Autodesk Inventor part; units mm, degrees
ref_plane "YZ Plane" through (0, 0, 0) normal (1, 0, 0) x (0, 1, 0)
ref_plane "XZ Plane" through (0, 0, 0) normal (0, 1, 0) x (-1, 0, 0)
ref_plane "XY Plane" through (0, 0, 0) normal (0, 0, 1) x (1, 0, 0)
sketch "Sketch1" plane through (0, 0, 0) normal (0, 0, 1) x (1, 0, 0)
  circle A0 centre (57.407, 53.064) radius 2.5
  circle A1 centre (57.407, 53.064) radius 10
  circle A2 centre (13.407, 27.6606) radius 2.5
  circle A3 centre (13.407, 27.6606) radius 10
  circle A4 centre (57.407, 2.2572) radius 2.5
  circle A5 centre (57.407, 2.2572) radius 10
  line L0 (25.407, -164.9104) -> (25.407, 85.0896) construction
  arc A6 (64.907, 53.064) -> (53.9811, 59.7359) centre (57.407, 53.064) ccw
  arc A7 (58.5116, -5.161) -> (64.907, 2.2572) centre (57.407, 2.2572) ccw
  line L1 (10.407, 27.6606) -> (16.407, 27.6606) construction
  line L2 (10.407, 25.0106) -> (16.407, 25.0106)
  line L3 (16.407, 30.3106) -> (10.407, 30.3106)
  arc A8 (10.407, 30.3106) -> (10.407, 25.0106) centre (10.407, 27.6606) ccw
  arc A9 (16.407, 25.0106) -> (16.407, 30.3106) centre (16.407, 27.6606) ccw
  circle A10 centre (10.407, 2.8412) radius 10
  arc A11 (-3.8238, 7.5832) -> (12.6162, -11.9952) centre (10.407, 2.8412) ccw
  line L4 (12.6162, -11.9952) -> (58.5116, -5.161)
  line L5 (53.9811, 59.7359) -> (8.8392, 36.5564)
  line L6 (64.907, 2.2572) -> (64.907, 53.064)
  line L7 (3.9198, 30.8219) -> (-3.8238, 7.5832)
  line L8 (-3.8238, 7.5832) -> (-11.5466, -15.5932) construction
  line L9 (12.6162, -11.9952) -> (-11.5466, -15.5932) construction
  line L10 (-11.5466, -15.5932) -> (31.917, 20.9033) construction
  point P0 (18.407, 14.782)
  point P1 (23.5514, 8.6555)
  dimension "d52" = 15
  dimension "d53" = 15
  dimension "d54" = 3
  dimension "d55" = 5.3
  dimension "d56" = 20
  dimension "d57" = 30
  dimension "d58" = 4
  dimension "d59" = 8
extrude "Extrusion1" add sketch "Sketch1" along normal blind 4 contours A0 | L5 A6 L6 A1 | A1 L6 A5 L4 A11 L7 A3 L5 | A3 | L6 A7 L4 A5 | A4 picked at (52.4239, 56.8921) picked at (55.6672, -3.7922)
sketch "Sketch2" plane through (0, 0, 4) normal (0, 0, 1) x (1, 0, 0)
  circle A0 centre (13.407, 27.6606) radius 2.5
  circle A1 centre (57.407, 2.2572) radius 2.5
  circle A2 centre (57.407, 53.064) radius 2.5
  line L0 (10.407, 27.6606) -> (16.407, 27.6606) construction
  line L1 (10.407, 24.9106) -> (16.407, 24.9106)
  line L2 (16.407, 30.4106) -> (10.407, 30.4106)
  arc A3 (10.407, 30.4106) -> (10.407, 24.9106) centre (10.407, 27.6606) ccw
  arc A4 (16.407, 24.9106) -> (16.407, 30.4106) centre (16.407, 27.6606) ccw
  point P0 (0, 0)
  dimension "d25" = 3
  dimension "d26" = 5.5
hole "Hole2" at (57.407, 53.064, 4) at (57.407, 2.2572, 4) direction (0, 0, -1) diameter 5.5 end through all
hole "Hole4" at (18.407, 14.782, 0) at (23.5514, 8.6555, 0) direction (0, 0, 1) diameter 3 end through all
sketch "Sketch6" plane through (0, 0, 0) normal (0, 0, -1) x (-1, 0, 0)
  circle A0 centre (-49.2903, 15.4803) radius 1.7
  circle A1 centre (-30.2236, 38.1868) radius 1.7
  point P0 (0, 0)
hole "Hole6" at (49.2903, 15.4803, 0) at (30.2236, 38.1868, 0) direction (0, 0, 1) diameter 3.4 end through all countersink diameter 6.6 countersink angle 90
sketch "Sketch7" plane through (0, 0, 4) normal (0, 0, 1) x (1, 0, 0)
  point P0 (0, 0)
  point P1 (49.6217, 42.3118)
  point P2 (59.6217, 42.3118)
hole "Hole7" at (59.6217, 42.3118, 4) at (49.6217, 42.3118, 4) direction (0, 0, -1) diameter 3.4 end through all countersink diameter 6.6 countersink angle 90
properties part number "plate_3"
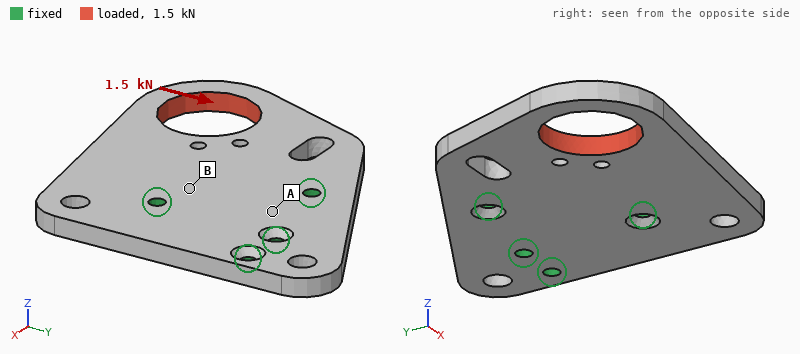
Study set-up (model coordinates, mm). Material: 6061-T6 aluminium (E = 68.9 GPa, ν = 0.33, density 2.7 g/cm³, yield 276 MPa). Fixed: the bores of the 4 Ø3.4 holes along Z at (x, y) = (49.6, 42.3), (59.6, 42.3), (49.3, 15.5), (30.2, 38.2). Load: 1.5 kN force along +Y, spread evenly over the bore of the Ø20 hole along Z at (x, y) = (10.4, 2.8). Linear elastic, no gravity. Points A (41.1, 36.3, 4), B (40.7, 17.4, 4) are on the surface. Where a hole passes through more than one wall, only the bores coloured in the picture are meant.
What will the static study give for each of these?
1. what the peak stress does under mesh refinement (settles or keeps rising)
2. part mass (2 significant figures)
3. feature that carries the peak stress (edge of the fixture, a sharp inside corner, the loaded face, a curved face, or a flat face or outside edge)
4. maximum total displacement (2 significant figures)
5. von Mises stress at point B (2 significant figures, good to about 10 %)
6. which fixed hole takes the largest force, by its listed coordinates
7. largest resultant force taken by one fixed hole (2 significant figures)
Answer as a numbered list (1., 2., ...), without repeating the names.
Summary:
1. keeps rising
2. 35 g
3. edge of the fixture
4. 52 µm
5. 18 MPa
6. (30.2, 38.2)
7. 1.6 kN
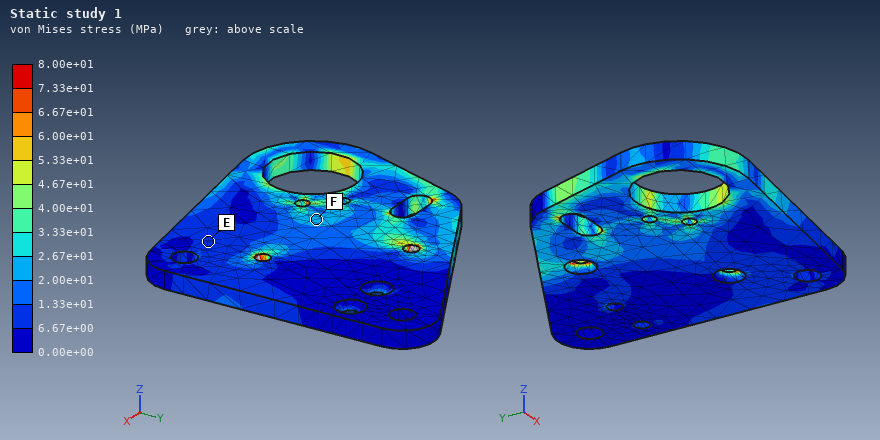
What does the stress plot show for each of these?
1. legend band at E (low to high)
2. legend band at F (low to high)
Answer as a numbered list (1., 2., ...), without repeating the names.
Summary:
1. 6.67e+00 to 1.33e+01 MPa
2. 2.00e+01 to 2.67e+01 MPa
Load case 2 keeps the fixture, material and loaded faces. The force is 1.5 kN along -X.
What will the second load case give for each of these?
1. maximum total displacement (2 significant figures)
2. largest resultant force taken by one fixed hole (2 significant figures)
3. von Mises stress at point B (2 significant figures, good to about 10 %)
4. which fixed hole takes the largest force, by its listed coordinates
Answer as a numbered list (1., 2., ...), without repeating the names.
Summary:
1. 41 µm
2. 1.6 kN
3. 21 MPa
4. (49.3, 15.5)
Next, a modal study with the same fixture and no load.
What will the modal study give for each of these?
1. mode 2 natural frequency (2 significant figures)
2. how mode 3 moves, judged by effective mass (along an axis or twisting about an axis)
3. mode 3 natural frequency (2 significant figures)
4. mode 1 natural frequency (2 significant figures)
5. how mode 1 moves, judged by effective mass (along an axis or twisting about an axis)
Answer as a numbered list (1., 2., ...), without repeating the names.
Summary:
1. 4000 Hz
2. along Z
3. 6100 Hz
4. 1700 Hz
5. along Z
